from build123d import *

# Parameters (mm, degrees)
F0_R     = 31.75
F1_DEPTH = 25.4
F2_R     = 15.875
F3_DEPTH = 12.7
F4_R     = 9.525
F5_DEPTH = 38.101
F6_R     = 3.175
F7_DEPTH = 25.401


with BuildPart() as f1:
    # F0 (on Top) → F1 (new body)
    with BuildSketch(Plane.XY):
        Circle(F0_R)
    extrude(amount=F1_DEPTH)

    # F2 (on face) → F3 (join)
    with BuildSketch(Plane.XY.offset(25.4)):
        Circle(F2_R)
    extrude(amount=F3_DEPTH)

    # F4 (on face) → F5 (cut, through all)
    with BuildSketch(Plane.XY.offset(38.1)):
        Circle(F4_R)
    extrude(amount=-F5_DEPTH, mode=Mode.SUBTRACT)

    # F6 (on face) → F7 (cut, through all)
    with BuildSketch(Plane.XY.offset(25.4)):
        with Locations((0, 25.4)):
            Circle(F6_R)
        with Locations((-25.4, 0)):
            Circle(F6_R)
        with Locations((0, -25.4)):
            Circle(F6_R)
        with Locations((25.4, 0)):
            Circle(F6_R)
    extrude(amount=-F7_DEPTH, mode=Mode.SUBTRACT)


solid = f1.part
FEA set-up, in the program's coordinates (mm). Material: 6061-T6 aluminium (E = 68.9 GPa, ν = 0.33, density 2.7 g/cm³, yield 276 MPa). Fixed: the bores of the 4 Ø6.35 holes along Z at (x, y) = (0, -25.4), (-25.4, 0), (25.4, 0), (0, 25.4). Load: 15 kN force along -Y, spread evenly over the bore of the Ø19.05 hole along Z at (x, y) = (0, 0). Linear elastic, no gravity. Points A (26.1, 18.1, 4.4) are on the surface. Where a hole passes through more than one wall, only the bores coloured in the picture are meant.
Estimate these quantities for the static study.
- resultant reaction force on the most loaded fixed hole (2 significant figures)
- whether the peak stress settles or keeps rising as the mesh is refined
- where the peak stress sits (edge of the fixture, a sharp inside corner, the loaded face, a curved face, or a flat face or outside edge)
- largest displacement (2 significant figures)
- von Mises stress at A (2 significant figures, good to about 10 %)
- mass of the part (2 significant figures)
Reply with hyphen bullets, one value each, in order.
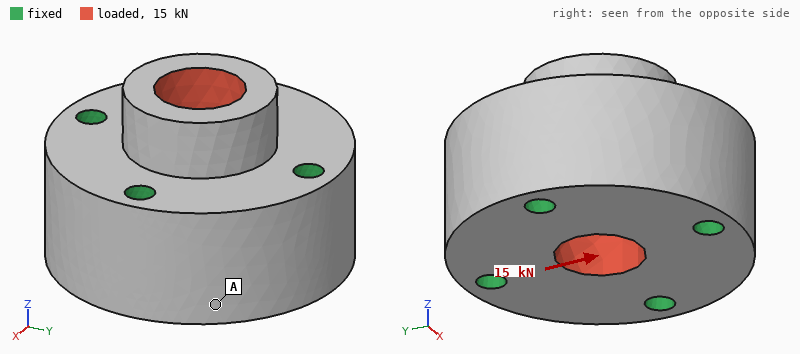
- 4.9 kN
- keeps rising
- a sharp inside corner
- 12 µm
- 3.5 MPa
- 210 g
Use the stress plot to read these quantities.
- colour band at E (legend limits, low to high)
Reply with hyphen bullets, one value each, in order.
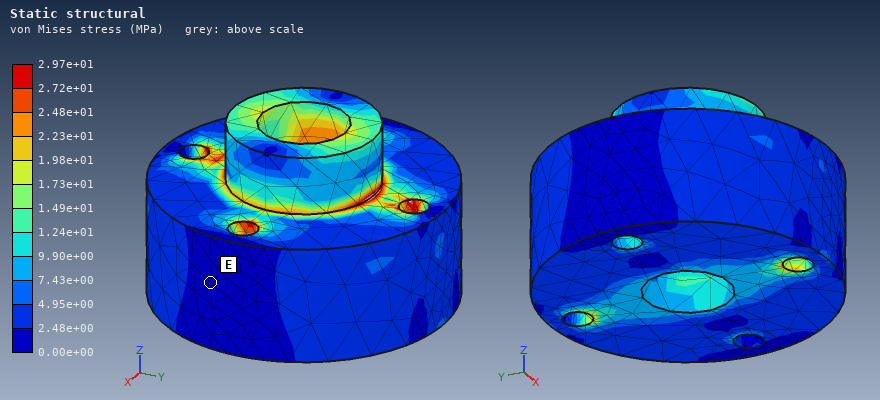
- 0.00e+00 to 2.48e+00 MPa
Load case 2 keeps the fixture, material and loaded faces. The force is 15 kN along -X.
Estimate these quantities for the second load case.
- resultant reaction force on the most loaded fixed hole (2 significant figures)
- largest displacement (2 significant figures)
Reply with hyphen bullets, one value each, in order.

- 4.9 kN
- 12 µm
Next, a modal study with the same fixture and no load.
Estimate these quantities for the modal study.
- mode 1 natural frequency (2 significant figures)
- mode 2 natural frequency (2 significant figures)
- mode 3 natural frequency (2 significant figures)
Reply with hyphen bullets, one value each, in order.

- 29 kHz
- 29 kHz
- 31 kHz
